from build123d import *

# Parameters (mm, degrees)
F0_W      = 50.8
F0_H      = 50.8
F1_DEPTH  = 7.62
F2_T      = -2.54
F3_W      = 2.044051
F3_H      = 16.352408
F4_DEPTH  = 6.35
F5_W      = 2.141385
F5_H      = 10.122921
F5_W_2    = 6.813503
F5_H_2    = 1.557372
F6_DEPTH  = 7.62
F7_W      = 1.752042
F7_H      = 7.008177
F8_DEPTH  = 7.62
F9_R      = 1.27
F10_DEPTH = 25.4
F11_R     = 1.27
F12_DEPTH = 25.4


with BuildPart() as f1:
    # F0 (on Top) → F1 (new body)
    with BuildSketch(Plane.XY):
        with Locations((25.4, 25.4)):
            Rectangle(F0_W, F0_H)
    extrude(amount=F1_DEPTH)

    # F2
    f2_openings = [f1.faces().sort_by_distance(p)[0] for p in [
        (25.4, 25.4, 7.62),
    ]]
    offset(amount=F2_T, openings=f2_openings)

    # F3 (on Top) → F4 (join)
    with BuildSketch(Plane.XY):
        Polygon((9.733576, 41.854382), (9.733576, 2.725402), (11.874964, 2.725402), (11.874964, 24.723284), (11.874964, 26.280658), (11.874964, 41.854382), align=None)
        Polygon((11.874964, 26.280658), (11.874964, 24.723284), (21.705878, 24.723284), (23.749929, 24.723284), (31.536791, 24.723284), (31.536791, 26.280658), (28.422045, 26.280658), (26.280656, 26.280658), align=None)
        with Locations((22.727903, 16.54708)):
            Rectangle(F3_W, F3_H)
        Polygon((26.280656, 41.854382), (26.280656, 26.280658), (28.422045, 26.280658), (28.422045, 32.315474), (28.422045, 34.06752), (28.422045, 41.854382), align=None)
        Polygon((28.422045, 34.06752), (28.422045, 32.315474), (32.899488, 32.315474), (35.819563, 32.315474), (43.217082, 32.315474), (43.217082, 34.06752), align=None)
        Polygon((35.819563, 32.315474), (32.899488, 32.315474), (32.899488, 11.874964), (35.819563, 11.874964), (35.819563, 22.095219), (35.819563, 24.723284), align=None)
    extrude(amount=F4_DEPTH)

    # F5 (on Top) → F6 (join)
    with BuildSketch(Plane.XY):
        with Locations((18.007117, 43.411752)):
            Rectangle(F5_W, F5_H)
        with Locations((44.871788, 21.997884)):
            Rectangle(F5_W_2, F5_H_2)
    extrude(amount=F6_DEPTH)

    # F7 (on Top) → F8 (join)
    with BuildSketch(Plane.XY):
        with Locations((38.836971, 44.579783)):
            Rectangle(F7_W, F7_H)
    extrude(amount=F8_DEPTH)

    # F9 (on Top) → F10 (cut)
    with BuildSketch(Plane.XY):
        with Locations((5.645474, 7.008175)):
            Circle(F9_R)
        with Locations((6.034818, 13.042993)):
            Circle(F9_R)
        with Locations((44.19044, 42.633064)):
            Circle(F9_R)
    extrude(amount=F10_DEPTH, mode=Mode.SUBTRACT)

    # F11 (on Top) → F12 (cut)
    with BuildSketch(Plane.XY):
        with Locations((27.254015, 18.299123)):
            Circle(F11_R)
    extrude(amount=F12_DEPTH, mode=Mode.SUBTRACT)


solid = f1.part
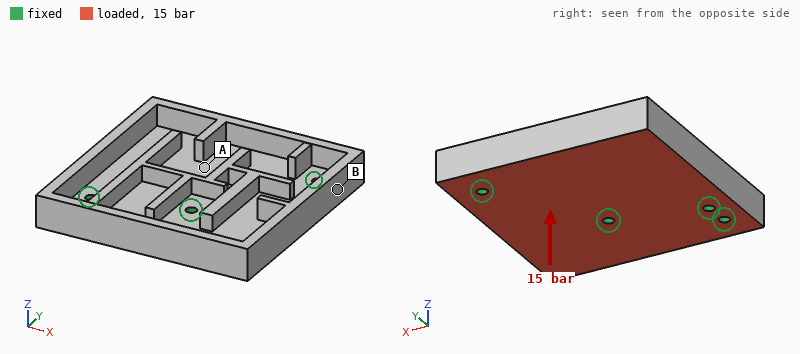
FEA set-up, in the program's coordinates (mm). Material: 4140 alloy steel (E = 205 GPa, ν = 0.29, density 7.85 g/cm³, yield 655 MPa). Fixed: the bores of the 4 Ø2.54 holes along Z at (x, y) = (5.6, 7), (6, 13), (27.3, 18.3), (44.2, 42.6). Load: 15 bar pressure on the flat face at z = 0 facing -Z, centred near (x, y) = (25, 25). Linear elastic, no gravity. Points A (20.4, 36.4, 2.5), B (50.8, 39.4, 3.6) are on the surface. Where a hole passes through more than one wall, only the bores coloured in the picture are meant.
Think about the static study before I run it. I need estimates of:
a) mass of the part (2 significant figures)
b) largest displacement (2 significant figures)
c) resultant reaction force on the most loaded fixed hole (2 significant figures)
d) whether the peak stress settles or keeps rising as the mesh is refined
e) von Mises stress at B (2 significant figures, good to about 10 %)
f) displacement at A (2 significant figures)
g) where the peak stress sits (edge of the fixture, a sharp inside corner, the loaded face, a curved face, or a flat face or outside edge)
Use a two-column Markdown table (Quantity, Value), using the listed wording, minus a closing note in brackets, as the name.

| Quantity | Value |
|---|---|
| mass of the part | 80 g |
| largest displacement | 0.17 mm |
| resultant reaction force on the most loaded fixed hole | 1.9 kN |
| whether the peak stress settles or keeps rising as the mesh is refined | keeps rising |
| von Mises stress at B | 87 MPa |
| displacement at A | 0.053 mm |
| where the peak stress sits | edge of the fixture |
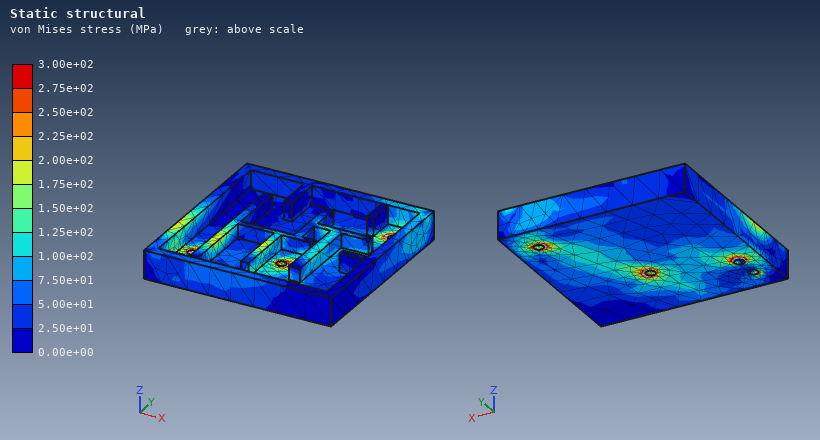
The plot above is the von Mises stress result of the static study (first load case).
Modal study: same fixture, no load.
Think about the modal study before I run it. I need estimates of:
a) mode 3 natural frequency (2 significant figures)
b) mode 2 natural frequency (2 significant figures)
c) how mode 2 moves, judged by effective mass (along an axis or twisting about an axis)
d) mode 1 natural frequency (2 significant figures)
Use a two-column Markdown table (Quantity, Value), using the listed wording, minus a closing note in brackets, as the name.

| Quantity | Value |
|---|---|
| mode 3 natural frequency | 11 kHz |
| mode 2 natural frequency | 4100 Hz |
| how mode 2 moves, judged by effective mass | along Z |
| mode 1 natural frequency | 3100 Hz |
